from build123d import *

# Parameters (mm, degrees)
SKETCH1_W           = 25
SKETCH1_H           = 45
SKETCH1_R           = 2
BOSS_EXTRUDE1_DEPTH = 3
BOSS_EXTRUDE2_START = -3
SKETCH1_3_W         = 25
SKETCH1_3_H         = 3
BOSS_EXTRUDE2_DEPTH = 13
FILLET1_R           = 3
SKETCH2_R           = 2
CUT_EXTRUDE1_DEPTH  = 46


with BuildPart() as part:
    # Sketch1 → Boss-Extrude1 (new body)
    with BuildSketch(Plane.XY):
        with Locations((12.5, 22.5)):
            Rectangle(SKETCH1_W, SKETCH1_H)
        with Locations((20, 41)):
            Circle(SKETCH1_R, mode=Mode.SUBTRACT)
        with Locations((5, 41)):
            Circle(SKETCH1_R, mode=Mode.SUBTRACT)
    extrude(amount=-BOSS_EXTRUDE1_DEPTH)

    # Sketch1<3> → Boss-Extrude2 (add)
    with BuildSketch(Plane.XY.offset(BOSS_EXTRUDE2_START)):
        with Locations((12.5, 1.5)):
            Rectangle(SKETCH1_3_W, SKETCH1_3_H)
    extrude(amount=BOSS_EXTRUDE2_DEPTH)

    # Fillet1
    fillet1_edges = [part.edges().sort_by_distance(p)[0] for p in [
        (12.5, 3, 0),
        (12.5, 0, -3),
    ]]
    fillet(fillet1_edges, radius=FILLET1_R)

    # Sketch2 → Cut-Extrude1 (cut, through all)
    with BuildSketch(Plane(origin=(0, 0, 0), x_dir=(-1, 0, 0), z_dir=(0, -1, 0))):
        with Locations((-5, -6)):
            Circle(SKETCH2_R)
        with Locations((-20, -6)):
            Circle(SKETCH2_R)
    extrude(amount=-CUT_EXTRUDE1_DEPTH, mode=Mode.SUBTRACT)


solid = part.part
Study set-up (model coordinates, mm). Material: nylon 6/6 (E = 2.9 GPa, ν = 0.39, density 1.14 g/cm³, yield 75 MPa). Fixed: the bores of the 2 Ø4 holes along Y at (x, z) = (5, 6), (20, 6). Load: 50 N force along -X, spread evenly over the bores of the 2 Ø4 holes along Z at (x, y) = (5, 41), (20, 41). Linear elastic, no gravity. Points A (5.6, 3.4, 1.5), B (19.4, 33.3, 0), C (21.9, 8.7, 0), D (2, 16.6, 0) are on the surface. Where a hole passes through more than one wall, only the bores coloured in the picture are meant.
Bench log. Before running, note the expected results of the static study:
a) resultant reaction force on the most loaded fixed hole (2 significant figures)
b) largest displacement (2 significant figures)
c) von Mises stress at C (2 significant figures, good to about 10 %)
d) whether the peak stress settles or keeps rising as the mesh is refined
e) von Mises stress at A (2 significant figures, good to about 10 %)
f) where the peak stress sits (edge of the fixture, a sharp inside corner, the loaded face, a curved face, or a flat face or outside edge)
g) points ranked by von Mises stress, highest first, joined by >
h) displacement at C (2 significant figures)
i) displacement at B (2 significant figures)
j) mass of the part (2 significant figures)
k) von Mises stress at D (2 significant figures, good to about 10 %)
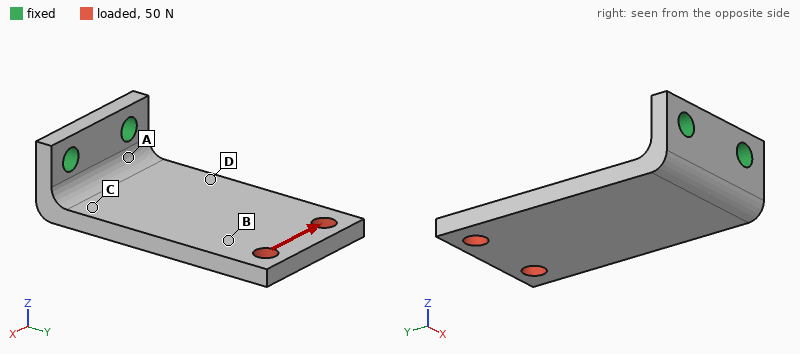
120 N
0.61 mm
9.5 MPa
keeps rising
14 MPa
edge of the fixture
A > C > D > B
0.15 mm
0.43 mm
4.5 g
5.0 MPa
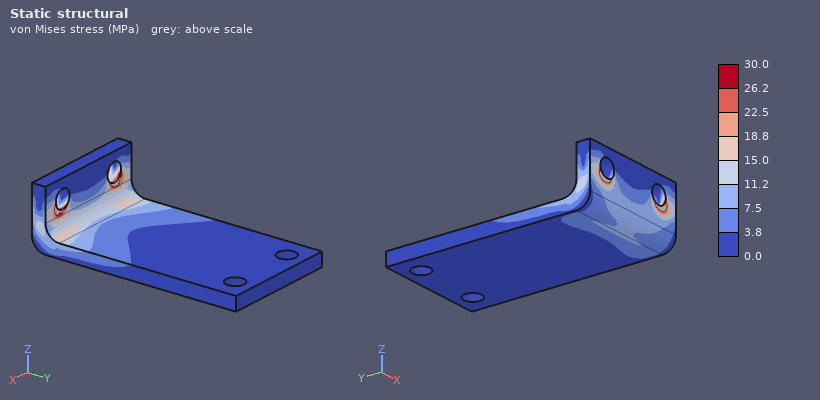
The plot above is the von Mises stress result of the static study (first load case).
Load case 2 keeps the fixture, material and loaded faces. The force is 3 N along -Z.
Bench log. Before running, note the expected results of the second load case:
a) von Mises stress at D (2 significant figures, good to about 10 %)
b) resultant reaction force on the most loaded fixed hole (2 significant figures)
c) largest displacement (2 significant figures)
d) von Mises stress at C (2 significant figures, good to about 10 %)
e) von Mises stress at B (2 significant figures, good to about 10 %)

1.9 MPa
2.5 N
0.49 mm
2.3 MPa
0.66 MPa
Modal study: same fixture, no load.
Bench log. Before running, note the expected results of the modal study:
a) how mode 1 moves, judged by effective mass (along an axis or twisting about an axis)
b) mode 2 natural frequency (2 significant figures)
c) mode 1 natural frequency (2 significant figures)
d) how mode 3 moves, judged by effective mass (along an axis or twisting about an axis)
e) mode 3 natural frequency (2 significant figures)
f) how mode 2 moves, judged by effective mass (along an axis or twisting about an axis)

along Z
1200 Hz
390 Hz
along X
1700 Hz
along X
